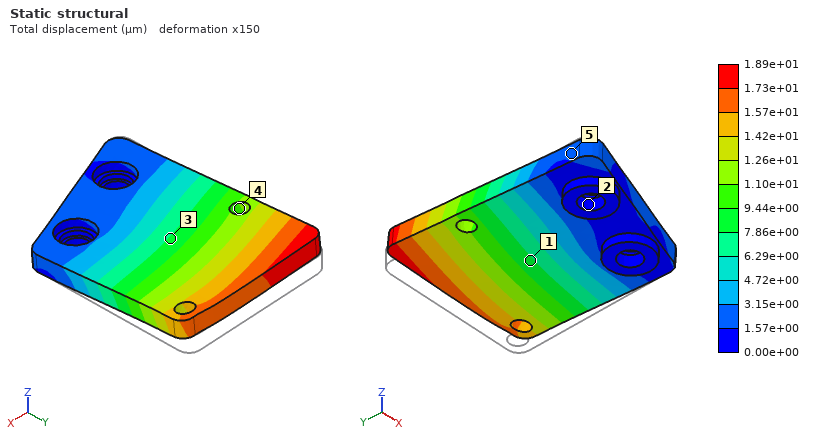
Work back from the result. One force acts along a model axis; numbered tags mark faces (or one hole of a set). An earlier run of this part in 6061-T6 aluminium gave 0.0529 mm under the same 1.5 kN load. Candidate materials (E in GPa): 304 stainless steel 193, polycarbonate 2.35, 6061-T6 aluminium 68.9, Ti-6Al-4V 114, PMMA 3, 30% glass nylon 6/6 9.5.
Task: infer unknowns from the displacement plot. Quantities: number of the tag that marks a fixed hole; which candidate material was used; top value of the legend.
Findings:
2
304 stainless steel
1.89e+01 µm
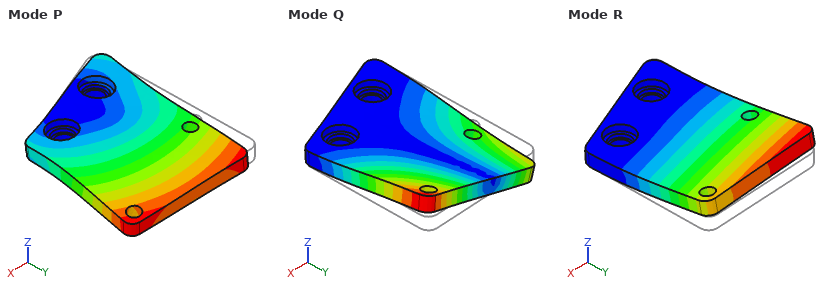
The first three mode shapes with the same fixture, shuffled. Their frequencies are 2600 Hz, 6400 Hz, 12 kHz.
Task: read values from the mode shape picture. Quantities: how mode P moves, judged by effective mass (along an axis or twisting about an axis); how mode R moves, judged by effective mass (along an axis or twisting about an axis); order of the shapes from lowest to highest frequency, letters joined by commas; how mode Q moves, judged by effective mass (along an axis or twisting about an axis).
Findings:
along X
along Z
R, Q, P
twisting about Y
